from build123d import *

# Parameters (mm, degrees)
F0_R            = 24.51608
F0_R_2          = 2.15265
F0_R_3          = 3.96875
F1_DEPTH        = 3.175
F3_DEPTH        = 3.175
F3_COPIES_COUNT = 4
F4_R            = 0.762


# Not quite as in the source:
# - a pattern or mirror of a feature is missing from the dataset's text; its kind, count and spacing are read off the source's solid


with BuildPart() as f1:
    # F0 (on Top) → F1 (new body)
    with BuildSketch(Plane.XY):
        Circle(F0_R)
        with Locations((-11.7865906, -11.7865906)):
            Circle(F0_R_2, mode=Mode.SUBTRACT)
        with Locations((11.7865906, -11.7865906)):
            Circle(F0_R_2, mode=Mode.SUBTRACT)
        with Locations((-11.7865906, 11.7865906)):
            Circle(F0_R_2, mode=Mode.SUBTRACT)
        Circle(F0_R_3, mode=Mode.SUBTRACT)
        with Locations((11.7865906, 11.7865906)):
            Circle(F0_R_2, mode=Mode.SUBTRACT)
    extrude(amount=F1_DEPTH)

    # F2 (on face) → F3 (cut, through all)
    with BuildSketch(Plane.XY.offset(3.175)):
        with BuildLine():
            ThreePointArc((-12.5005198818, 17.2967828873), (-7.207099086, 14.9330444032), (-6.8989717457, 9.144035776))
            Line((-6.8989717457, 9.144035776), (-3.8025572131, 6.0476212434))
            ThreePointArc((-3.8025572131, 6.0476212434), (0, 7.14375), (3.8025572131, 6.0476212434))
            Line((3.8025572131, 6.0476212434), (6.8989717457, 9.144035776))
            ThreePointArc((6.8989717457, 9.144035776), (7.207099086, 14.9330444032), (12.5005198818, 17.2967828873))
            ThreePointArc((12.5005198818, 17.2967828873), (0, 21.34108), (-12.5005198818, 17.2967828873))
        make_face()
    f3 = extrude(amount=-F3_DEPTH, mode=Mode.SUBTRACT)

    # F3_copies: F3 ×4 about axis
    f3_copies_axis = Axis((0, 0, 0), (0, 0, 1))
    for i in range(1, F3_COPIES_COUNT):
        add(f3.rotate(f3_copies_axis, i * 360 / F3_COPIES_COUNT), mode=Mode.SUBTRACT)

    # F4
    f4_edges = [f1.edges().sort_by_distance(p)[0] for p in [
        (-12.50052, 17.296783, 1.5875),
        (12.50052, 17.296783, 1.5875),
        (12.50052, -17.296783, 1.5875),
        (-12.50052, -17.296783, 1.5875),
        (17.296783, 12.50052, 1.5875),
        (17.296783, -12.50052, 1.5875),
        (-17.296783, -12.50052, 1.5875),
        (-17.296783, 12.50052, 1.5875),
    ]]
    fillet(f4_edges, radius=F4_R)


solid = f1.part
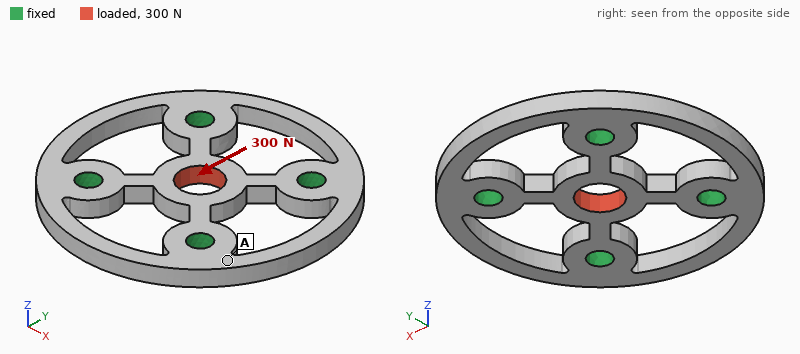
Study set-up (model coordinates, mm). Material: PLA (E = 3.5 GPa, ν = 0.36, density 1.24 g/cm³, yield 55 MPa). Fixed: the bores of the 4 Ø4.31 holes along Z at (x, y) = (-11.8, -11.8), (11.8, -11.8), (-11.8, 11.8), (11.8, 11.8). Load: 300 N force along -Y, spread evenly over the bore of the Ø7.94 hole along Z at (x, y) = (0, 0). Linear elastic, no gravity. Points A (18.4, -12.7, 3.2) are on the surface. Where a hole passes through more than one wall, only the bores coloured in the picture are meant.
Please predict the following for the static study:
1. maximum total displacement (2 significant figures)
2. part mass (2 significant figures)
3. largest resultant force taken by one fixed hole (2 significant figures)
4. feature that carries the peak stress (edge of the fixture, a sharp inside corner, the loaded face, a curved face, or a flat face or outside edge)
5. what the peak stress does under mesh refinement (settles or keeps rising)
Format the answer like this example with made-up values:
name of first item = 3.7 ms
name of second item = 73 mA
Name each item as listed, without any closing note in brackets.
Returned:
maximum total displacement = 51 µm
part mass = 3.7 g
largest resultant force taken by one fixed hole = 92 N
feature that carries the peak stress = a sharp inside corner
what the peak stress does under mesh refinement = keeps rising
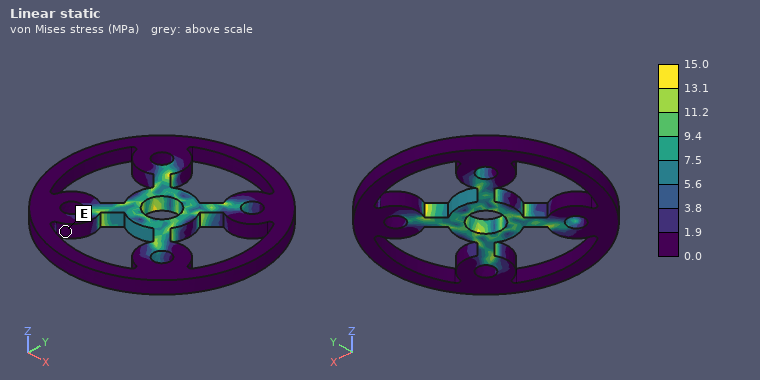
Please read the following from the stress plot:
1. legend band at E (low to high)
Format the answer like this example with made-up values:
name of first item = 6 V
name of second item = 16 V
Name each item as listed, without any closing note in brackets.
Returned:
legend band at E = 0.0 to 1.9 MPa
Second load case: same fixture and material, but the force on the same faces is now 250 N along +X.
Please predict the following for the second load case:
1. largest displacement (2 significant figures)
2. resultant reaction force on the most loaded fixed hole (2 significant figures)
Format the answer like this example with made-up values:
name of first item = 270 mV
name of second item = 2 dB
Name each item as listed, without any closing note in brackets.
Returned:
largest displacement = 42 µm
resultant reaction force on the most loaded fixed hole = 77 N
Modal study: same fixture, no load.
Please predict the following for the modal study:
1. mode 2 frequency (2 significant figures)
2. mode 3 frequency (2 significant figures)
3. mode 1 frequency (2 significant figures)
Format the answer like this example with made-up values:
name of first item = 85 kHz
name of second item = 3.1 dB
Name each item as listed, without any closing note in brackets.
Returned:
mode 2 frequency = 4400 Hz
mode 3 frequency = 4400 Hz
mode 1 frequency = 4100 Hz
